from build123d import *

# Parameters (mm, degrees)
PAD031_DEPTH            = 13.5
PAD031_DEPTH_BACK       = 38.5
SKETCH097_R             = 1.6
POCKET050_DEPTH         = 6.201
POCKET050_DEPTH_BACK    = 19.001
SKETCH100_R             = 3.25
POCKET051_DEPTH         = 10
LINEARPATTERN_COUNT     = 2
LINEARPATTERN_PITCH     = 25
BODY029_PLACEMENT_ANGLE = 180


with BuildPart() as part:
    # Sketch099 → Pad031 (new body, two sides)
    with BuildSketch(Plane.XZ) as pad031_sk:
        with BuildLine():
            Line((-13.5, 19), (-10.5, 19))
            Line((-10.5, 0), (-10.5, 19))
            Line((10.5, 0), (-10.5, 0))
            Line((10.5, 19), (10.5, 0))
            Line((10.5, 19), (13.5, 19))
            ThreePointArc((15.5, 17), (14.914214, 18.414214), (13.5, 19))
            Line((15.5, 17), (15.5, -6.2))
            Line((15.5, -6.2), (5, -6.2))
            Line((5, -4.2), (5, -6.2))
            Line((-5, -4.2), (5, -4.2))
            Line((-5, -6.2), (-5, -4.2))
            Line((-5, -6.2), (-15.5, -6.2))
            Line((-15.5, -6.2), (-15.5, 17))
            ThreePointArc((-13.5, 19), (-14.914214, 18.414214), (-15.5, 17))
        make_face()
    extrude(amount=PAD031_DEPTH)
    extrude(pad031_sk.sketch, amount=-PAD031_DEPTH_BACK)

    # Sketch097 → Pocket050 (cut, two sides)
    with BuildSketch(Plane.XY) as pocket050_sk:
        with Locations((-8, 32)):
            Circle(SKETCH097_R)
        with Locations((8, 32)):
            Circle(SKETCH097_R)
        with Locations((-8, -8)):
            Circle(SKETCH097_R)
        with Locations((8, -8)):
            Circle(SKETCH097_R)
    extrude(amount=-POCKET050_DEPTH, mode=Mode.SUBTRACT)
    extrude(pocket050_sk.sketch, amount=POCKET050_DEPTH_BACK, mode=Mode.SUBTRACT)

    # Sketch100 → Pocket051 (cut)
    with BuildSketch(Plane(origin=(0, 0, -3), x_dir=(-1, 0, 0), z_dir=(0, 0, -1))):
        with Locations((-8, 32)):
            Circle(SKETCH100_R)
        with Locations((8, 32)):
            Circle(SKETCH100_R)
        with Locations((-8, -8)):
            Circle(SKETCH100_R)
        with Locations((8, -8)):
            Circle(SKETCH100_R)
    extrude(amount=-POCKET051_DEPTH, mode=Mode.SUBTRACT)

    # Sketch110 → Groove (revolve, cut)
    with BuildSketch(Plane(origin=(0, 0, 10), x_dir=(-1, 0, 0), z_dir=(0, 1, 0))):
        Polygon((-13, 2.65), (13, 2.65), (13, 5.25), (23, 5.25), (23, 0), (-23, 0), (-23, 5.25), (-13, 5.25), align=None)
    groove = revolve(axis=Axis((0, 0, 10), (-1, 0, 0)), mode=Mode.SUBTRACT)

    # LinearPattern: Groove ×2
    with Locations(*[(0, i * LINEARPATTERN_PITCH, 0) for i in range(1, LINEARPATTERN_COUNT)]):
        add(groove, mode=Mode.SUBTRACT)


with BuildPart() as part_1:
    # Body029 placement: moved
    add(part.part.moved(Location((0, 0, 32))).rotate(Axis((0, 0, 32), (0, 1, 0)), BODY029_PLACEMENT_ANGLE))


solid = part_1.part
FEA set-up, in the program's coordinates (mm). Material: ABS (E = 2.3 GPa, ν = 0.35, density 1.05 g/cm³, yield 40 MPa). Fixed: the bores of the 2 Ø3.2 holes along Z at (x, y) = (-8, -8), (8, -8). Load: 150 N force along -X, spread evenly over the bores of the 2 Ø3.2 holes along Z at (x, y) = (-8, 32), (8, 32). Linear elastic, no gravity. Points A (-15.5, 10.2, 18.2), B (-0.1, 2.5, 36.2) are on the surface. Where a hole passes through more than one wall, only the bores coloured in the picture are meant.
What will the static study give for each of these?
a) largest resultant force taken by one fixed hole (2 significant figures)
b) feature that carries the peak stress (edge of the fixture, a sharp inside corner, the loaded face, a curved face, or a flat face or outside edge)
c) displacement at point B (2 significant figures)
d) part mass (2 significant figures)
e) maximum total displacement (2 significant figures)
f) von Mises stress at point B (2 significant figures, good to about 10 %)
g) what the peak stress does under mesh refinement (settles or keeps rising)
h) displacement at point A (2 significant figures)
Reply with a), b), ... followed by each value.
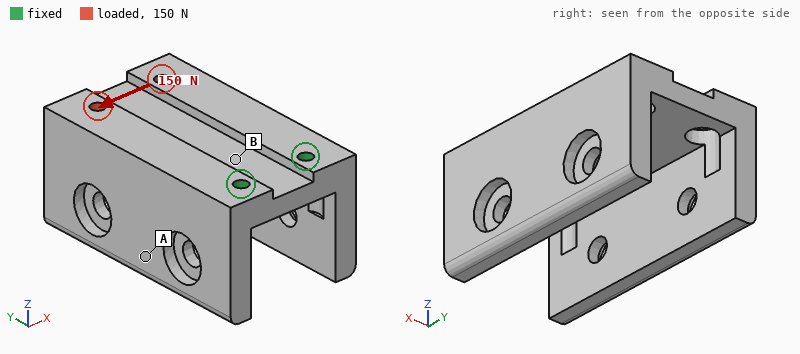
a) 330 N
b) edge of the fixture
c) 0.064 mm
d) 18 g
e) 0.41 mm
f) 6.2 MPa
g) keeps rising
h) 0.17 mm
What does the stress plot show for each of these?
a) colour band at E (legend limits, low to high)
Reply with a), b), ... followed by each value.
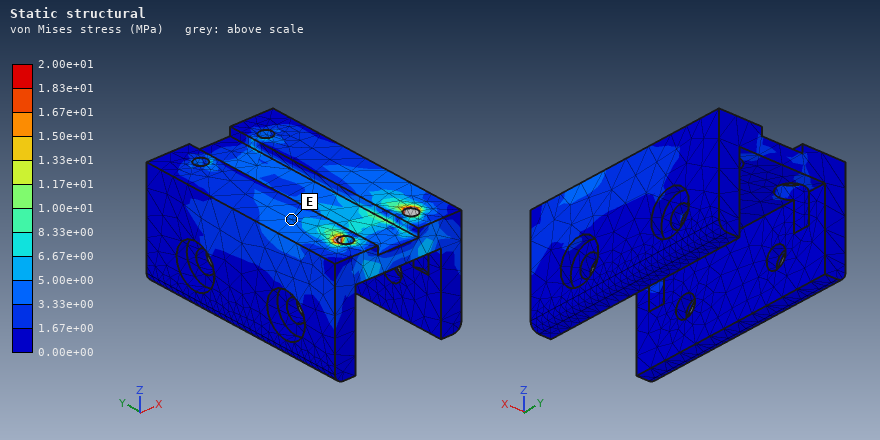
a) 3.33e+00 to 5.00e+00 MPa
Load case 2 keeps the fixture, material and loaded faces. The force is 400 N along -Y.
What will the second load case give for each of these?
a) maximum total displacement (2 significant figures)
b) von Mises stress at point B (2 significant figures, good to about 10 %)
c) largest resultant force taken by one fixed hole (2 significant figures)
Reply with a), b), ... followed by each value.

a) 0.15 mm
b) 2.7 MPa
c) 200 N
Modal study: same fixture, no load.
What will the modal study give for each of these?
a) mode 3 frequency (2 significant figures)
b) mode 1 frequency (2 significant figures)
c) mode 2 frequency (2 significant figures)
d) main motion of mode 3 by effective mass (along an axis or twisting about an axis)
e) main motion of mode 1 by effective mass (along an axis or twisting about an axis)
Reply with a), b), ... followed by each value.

a) 1300 Hz
b) 440 Hz
c) 850 Hz
d) along X
e) along Z
